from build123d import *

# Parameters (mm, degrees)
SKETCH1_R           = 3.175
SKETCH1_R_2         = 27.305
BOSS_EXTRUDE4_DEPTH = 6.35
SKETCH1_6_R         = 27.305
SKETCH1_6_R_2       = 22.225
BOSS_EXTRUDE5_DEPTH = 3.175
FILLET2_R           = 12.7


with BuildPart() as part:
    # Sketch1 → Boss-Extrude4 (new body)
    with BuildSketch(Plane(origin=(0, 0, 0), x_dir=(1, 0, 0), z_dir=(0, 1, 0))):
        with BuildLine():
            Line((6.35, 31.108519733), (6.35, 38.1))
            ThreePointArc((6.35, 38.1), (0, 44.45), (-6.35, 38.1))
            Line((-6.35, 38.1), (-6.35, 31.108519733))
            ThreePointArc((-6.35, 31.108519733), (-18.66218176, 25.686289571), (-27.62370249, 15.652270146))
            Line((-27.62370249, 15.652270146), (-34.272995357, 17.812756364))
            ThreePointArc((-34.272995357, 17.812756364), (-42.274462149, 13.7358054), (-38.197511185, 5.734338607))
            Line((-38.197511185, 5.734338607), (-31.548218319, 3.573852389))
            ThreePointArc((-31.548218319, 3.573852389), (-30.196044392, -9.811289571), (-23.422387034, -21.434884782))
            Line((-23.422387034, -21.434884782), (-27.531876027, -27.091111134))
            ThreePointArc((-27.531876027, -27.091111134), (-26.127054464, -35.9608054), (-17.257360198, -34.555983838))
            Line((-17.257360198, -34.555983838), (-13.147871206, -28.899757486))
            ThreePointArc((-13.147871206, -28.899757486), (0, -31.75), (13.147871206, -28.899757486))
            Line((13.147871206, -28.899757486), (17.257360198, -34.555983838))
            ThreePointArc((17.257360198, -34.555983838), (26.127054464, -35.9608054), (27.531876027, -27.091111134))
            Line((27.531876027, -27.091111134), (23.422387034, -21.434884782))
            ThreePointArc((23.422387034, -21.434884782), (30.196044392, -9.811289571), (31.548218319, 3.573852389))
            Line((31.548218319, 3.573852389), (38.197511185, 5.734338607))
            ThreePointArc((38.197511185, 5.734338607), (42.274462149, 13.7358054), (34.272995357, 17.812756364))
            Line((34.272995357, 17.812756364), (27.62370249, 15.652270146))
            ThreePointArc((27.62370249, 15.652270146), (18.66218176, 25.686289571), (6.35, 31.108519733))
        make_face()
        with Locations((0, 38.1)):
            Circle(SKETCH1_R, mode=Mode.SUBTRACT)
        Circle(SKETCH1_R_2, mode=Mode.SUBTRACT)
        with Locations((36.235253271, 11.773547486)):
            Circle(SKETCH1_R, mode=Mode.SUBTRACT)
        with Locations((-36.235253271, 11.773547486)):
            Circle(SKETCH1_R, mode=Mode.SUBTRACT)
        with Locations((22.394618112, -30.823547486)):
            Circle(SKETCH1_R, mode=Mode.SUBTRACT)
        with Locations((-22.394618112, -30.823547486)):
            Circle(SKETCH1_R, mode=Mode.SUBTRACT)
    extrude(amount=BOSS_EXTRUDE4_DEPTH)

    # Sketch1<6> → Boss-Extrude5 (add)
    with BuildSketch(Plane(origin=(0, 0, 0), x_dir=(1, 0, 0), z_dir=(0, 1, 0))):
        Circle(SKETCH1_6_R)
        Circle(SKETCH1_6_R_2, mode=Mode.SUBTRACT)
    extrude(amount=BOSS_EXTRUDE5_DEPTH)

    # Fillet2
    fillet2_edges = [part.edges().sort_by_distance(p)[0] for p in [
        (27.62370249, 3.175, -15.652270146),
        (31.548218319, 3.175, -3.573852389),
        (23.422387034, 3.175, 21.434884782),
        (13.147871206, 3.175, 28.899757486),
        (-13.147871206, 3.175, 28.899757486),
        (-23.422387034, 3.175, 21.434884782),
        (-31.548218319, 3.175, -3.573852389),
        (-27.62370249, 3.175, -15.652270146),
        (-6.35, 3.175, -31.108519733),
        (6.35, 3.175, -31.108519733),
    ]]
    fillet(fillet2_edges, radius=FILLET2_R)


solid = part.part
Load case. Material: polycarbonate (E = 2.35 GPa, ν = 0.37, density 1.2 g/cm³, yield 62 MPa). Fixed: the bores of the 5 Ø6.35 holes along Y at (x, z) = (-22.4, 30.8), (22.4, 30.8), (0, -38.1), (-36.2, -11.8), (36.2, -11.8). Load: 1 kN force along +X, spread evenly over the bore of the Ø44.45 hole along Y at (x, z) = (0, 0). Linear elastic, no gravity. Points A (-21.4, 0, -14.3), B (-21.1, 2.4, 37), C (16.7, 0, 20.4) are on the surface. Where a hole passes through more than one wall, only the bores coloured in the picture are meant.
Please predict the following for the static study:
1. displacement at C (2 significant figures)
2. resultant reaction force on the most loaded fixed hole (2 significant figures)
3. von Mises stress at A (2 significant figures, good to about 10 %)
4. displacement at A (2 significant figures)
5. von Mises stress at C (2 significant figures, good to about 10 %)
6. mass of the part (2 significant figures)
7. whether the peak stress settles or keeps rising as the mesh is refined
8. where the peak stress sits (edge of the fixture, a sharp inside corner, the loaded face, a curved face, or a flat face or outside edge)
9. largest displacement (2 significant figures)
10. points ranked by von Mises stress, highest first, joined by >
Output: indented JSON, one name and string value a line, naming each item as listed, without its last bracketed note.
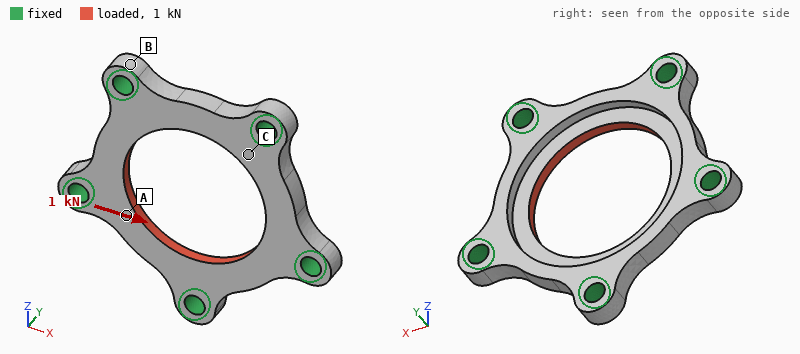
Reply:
{
  "displacement at C": "31 µm",
  "resultant reaction force on the most loaded fixed hole": "260 N",
  "von Mises stress at A": "5.1 MPa",
  "displacement at A": "29 µm",
  "von Mises stress at C": "2.8 MPa",
  "mass of the part": "15 g",
  "whether the peak stress settles or keeps rising as the mesh is refined": "keeps rising",
  "where the peak stress sits": "edge of the fixture",
  "largest displacement": "81 µm",
  "points ranked by von Mises stress, highest first, joined by >": "A > C > B"
}
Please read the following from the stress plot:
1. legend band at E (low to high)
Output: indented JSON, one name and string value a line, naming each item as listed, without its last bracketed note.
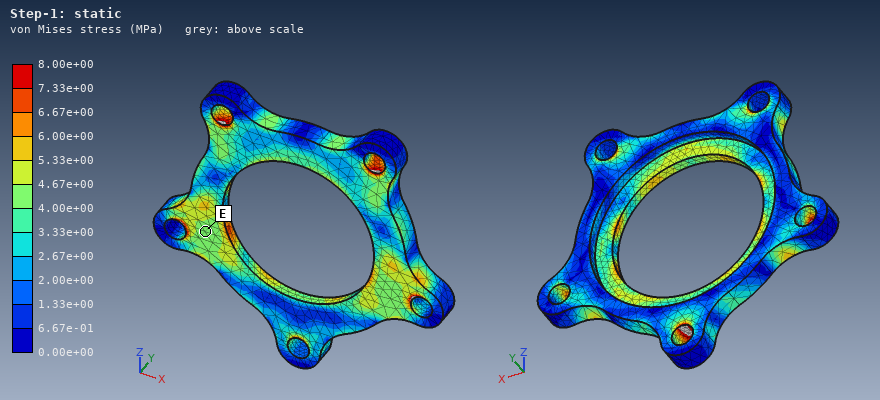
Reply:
{
  "legend band at E": "4.00e+00 to 4.67e+00 MPa"
}
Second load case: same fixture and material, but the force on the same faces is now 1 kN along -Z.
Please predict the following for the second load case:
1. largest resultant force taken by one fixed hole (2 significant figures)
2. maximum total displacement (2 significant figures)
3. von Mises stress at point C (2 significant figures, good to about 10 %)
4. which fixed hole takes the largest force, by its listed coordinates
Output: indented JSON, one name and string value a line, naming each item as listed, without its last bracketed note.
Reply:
{
  "largest resultant force taken by one fixed hole": "270 N",
  "maximum total displacement": "85 µm",
  "von Mises stress at point C": "3.5 MPa",
  "which fixed hole takes the largest force, by its listed coordinates": "(0, -38.1)"
}
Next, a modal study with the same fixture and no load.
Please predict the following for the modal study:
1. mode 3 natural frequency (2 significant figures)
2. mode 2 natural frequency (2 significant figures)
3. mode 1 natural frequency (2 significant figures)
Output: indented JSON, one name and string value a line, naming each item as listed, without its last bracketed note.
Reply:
{
  "mode 3 natural frequency": "5000 Hz",
  "mode 2 natural frequency": "5000 Hz",
  "mode 1 natural frequency": "4900 Hz"
}
